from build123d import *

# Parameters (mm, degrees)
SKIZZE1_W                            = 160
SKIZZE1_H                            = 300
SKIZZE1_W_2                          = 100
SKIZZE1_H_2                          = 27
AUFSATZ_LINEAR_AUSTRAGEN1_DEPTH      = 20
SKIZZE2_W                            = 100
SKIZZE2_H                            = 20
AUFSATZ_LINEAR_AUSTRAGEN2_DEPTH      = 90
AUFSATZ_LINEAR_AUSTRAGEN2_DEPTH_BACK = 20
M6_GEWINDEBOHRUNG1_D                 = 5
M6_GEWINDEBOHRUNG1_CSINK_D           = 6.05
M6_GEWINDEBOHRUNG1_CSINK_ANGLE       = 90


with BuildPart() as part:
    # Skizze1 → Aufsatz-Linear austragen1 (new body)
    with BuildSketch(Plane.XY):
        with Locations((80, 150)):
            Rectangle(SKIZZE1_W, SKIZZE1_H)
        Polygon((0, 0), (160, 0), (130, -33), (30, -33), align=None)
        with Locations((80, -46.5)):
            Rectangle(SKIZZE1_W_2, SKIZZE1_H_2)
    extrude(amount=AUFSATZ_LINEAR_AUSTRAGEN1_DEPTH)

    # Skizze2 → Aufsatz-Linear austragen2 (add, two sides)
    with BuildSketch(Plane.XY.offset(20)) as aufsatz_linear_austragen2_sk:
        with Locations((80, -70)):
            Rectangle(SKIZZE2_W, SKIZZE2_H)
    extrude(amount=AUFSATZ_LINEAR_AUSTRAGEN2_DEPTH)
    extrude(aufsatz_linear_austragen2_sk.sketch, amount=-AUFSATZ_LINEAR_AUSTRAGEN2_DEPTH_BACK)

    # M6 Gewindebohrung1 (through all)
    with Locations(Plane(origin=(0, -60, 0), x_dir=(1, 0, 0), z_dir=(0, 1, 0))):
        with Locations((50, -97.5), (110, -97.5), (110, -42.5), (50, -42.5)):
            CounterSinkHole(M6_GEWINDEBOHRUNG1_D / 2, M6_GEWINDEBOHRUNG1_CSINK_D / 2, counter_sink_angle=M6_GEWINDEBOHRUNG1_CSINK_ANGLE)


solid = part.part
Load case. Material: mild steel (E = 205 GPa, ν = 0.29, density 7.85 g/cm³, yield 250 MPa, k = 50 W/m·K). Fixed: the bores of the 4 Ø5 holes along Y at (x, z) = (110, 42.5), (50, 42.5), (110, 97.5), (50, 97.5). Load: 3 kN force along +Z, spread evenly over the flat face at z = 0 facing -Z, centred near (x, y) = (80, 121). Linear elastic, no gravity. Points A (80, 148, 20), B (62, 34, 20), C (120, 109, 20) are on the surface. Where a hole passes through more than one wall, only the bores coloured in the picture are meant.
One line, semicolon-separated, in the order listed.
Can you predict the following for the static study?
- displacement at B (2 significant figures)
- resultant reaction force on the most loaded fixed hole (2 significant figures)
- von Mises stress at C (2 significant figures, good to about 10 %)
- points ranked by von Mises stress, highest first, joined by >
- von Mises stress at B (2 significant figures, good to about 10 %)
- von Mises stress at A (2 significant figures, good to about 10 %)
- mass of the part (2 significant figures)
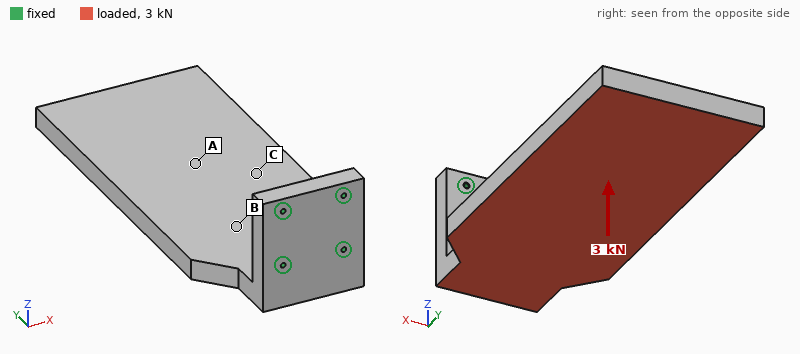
0.31 mm; 2.9 kN; 14 MPa; B > C > A; 28 MPa; 9.2 MPa; 10 kg
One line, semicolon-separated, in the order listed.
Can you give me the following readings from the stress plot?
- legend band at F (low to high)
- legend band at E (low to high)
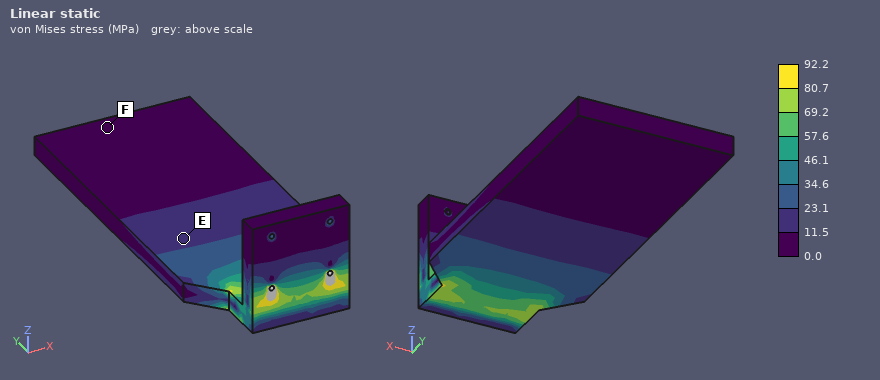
0.0 to 11.5 MPa; 11.5 to 23.1 MPa
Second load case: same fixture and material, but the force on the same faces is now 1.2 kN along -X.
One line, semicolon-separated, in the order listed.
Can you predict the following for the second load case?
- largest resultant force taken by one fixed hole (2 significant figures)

3.5 kN
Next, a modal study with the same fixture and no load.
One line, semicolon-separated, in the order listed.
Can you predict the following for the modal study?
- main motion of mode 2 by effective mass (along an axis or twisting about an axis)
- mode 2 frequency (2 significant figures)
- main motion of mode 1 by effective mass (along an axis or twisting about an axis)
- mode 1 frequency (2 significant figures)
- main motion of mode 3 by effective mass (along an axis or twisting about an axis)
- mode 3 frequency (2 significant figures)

along X; 260 Hz; along Z; 89 Hz; twisting about Y; 500 Hz
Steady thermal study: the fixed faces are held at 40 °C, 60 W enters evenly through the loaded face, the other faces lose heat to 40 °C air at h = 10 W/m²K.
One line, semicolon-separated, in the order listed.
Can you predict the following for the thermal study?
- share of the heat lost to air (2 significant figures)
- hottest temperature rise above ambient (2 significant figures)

49 %; 48 K
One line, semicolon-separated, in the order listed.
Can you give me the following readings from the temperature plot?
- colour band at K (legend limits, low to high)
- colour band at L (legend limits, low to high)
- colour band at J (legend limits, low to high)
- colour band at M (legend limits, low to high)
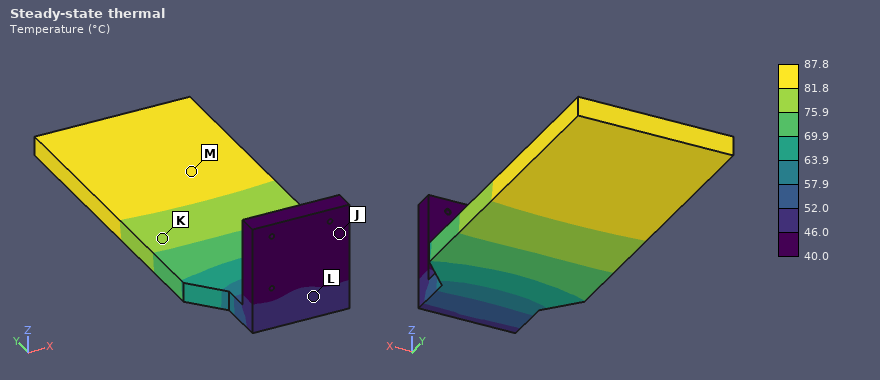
75.9 to 81.8 °C; 46.0 to 52.0 °C; 40.0 to 46.0 °C; 81.8 to 87.8 °C
